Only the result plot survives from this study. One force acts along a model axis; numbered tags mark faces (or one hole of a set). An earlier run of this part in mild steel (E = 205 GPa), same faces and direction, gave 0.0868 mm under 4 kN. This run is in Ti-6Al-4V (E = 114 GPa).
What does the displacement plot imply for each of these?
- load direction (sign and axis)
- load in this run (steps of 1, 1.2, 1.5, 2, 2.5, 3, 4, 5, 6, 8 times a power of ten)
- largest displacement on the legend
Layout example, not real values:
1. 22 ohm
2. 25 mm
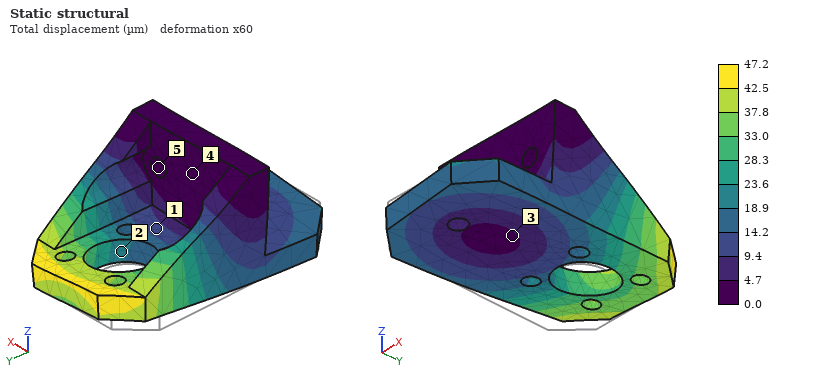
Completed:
1. +X
2. 1.2 kN
3. 47.2 µm
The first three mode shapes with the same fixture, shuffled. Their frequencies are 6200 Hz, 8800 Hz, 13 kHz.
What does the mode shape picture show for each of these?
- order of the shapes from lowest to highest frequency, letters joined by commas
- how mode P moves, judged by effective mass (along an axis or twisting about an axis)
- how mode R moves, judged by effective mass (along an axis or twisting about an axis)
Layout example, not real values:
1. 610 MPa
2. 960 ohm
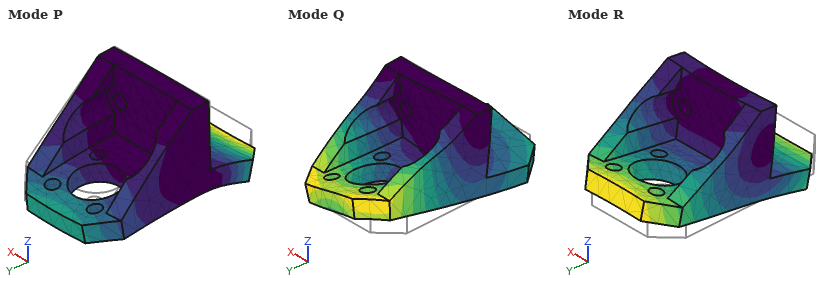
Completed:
1. R, Q, P
2. along Z
3. along Y
